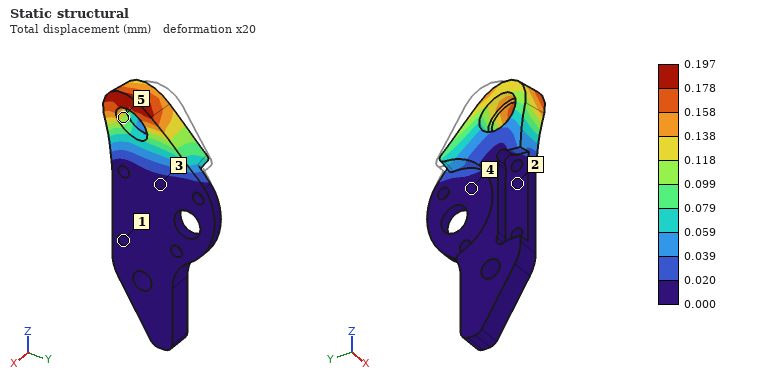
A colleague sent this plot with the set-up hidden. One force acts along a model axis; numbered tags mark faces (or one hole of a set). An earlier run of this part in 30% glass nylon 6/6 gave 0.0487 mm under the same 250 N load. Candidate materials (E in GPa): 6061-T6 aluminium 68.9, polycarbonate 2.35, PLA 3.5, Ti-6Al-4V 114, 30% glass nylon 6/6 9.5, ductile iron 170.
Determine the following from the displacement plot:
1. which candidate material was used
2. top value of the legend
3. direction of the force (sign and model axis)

polycarbonate
0.197 mm
-Y
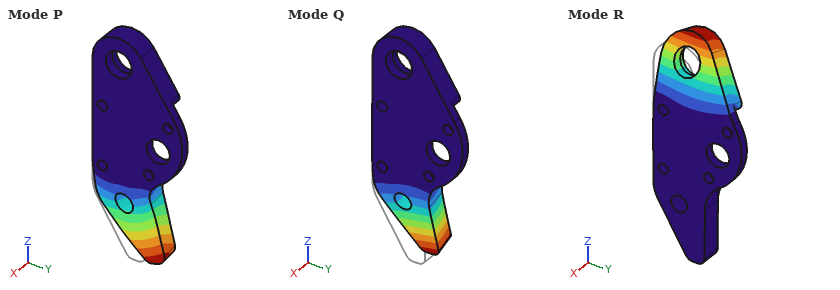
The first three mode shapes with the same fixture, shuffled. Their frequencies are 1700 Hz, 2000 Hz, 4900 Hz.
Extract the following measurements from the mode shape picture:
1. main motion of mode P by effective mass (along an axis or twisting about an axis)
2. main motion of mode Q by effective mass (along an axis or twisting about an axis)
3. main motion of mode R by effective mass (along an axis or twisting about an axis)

along Y
along X
along X
